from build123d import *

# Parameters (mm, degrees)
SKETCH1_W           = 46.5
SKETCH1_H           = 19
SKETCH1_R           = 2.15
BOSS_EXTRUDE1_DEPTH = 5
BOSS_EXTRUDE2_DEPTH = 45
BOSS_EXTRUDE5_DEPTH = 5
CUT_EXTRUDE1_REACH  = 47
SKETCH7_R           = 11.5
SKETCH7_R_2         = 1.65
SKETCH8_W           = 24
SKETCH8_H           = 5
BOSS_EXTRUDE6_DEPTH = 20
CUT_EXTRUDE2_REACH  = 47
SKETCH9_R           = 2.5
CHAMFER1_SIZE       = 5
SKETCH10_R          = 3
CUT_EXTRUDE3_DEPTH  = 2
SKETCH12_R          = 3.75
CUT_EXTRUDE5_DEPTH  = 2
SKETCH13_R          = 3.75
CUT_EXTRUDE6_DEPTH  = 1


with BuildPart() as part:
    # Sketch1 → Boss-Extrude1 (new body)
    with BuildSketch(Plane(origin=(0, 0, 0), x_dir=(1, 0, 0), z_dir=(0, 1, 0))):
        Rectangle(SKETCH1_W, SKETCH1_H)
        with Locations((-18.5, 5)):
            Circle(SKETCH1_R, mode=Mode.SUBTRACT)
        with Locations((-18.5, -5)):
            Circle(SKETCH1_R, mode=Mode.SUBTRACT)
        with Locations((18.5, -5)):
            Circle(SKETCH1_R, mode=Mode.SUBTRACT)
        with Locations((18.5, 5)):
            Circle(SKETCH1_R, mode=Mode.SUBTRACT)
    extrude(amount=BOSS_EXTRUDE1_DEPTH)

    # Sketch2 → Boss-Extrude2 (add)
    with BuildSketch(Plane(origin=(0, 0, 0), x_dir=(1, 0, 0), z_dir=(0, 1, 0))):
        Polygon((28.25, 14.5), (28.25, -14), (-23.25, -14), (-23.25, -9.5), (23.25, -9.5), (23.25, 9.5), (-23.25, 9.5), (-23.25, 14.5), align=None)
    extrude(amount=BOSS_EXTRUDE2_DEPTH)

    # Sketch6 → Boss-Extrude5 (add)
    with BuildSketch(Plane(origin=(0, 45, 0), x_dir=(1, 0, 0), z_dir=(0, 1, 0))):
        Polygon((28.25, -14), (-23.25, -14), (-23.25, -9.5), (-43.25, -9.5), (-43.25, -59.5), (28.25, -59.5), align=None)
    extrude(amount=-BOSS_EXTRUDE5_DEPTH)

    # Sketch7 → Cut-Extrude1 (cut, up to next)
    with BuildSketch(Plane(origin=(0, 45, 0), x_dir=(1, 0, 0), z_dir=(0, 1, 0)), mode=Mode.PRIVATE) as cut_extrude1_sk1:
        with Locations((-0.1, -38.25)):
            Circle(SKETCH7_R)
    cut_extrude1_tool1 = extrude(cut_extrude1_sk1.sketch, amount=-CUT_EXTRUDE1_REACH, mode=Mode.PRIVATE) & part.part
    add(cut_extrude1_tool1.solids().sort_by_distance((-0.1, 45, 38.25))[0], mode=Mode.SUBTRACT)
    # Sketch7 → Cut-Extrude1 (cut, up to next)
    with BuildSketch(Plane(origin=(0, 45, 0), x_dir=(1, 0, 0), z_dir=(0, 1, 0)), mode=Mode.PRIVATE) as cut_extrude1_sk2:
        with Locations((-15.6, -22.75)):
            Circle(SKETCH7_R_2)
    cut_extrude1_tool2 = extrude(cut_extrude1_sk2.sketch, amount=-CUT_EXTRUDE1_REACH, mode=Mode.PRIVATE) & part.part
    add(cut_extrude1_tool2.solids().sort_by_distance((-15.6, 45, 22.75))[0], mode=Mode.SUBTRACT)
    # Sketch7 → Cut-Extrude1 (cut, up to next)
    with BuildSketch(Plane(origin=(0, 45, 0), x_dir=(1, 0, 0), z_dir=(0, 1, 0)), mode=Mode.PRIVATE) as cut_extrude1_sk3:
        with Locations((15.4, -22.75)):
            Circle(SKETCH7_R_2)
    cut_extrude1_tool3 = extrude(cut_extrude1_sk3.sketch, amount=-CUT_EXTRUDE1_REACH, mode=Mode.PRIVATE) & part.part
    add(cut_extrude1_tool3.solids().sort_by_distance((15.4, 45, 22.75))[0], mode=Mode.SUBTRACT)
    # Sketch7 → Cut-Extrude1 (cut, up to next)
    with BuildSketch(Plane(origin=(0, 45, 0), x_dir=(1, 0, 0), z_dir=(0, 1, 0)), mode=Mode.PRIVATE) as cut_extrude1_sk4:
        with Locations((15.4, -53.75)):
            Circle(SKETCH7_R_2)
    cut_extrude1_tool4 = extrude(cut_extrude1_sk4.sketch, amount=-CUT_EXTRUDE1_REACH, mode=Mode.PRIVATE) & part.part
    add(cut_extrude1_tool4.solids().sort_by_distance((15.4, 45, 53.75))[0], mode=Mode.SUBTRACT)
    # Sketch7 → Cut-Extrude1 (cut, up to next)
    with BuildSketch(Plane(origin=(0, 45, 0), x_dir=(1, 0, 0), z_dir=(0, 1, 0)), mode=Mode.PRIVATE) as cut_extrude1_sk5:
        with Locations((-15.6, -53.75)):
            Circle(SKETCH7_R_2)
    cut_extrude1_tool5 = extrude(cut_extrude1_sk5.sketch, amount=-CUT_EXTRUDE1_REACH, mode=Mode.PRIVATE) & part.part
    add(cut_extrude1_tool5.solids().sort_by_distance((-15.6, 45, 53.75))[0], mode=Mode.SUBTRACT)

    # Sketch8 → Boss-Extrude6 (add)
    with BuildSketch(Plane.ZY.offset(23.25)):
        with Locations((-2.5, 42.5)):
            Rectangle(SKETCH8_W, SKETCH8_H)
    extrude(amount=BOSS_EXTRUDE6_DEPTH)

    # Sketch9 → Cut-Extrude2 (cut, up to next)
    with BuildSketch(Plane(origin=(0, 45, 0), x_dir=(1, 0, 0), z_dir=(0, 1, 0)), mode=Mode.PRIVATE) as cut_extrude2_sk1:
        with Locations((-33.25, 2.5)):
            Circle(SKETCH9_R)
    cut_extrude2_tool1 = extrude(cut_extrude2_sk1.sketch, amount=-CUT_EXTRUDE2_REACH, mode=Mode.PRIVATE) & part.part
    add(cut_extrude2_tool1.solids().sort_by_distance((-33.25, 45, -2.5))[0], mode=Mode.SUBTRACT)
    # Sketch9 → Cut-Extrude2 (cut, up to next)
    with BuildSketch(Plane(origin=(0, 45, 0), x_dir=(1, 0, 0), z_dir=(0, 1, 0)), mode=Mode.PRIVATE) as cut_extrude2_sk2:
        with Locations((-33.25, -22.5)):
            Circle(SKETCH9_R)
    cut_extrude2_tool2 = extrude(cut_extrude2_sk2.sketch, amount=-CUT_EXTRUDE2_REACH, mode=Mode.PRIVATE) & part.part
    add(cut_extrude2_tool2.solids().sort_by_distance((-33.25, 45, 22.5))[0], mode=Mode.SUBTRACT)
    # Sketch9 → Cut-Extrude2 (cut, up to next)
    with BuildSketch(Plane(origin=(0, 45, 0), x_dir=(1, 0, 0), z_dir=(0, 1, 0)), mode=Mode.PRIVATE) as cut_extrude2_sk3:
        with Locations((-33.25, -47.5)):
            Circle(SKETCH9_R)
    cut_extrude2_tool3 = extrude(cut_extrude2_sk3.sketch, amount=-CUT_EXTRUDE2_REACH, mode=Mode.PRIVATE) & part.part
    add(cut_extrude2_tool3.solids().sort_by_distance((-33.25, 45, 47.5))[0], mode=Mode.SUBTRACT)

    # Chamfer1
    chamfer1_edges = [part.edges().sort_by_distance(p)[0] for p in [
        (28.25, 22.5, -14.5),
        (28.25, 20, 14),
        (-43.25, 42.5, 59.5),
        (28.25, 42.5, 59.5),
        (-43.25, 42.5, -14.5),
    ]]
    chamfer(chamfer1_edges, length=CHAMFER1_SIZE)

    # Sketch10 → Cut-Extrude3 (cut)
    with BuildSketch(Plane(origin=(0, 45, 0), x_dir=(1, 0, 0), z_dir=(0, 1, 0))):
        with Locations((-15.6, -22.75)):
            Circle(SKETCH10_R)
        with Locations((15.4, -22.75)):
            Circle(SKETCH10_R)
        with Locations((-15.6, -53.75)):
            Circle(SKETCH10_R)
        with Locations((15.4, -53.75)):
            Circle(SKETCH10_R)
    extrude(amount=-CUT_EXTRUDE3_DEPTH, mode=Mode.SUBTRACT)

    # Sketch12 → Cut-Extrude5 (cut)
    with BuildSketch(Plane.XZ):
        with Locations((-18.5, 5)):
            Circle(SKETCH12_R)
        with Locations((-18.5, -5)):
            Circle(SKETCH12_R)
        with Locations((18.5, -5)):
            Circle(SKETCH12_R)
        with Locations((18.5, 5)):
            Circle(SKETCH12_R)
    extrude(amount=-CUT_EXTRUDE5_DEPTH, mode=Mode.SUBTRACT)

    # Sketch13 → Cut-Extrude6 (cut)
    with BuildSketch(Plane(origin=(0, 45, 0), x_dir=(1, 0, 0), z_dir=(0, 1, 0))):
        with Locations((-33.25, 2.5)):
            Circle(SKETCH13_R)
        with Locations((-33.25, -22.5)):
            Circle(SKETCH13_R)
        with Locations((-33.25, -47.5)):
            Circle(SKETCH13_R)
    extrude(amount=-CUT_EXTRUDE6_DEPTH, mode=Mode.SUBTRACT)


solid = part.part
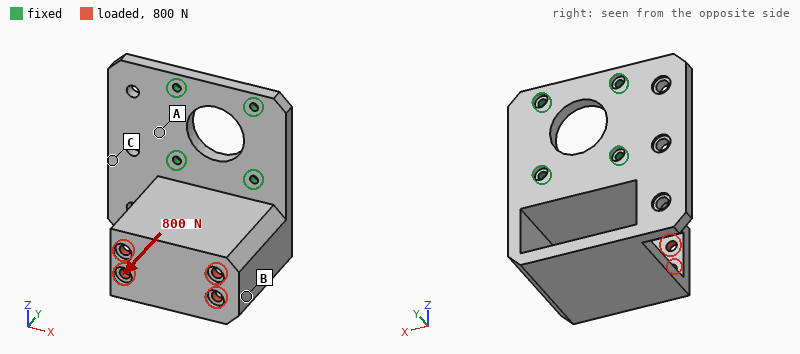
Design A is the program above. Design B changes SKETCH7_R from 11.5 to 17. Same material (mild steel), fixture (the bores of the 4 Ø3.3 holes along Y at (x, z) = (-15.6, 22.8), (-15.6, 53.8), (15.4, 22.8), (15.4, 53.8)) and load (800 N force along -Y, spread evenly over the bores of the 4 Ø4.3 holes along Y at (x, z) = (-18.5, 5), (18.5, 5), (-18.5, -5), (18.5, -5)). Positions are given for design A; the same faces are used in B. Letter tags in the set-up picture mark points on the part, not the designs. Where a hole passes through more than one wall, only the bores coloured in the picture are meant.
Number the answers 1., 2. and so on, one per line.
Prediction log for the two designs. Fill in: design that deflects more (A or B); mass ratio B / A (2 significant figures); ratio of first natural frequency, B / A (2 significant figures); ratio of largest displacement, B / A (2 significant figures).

1. B
2. 0.95
3. 0.94
4. 1.1
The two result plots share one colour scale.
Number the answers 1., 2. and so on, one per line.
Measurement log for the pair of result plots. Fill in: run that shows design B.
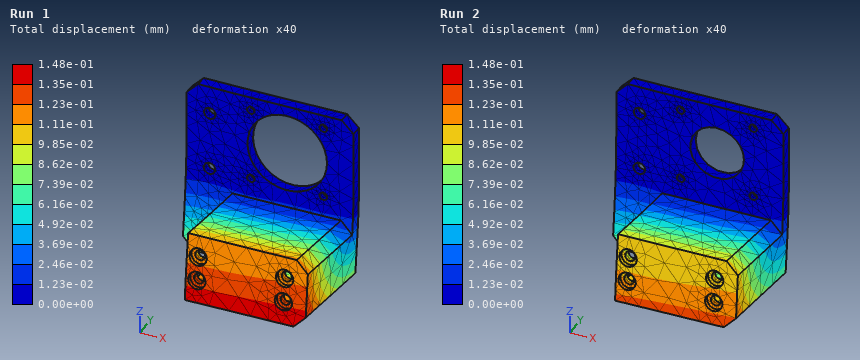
1. Run 1
